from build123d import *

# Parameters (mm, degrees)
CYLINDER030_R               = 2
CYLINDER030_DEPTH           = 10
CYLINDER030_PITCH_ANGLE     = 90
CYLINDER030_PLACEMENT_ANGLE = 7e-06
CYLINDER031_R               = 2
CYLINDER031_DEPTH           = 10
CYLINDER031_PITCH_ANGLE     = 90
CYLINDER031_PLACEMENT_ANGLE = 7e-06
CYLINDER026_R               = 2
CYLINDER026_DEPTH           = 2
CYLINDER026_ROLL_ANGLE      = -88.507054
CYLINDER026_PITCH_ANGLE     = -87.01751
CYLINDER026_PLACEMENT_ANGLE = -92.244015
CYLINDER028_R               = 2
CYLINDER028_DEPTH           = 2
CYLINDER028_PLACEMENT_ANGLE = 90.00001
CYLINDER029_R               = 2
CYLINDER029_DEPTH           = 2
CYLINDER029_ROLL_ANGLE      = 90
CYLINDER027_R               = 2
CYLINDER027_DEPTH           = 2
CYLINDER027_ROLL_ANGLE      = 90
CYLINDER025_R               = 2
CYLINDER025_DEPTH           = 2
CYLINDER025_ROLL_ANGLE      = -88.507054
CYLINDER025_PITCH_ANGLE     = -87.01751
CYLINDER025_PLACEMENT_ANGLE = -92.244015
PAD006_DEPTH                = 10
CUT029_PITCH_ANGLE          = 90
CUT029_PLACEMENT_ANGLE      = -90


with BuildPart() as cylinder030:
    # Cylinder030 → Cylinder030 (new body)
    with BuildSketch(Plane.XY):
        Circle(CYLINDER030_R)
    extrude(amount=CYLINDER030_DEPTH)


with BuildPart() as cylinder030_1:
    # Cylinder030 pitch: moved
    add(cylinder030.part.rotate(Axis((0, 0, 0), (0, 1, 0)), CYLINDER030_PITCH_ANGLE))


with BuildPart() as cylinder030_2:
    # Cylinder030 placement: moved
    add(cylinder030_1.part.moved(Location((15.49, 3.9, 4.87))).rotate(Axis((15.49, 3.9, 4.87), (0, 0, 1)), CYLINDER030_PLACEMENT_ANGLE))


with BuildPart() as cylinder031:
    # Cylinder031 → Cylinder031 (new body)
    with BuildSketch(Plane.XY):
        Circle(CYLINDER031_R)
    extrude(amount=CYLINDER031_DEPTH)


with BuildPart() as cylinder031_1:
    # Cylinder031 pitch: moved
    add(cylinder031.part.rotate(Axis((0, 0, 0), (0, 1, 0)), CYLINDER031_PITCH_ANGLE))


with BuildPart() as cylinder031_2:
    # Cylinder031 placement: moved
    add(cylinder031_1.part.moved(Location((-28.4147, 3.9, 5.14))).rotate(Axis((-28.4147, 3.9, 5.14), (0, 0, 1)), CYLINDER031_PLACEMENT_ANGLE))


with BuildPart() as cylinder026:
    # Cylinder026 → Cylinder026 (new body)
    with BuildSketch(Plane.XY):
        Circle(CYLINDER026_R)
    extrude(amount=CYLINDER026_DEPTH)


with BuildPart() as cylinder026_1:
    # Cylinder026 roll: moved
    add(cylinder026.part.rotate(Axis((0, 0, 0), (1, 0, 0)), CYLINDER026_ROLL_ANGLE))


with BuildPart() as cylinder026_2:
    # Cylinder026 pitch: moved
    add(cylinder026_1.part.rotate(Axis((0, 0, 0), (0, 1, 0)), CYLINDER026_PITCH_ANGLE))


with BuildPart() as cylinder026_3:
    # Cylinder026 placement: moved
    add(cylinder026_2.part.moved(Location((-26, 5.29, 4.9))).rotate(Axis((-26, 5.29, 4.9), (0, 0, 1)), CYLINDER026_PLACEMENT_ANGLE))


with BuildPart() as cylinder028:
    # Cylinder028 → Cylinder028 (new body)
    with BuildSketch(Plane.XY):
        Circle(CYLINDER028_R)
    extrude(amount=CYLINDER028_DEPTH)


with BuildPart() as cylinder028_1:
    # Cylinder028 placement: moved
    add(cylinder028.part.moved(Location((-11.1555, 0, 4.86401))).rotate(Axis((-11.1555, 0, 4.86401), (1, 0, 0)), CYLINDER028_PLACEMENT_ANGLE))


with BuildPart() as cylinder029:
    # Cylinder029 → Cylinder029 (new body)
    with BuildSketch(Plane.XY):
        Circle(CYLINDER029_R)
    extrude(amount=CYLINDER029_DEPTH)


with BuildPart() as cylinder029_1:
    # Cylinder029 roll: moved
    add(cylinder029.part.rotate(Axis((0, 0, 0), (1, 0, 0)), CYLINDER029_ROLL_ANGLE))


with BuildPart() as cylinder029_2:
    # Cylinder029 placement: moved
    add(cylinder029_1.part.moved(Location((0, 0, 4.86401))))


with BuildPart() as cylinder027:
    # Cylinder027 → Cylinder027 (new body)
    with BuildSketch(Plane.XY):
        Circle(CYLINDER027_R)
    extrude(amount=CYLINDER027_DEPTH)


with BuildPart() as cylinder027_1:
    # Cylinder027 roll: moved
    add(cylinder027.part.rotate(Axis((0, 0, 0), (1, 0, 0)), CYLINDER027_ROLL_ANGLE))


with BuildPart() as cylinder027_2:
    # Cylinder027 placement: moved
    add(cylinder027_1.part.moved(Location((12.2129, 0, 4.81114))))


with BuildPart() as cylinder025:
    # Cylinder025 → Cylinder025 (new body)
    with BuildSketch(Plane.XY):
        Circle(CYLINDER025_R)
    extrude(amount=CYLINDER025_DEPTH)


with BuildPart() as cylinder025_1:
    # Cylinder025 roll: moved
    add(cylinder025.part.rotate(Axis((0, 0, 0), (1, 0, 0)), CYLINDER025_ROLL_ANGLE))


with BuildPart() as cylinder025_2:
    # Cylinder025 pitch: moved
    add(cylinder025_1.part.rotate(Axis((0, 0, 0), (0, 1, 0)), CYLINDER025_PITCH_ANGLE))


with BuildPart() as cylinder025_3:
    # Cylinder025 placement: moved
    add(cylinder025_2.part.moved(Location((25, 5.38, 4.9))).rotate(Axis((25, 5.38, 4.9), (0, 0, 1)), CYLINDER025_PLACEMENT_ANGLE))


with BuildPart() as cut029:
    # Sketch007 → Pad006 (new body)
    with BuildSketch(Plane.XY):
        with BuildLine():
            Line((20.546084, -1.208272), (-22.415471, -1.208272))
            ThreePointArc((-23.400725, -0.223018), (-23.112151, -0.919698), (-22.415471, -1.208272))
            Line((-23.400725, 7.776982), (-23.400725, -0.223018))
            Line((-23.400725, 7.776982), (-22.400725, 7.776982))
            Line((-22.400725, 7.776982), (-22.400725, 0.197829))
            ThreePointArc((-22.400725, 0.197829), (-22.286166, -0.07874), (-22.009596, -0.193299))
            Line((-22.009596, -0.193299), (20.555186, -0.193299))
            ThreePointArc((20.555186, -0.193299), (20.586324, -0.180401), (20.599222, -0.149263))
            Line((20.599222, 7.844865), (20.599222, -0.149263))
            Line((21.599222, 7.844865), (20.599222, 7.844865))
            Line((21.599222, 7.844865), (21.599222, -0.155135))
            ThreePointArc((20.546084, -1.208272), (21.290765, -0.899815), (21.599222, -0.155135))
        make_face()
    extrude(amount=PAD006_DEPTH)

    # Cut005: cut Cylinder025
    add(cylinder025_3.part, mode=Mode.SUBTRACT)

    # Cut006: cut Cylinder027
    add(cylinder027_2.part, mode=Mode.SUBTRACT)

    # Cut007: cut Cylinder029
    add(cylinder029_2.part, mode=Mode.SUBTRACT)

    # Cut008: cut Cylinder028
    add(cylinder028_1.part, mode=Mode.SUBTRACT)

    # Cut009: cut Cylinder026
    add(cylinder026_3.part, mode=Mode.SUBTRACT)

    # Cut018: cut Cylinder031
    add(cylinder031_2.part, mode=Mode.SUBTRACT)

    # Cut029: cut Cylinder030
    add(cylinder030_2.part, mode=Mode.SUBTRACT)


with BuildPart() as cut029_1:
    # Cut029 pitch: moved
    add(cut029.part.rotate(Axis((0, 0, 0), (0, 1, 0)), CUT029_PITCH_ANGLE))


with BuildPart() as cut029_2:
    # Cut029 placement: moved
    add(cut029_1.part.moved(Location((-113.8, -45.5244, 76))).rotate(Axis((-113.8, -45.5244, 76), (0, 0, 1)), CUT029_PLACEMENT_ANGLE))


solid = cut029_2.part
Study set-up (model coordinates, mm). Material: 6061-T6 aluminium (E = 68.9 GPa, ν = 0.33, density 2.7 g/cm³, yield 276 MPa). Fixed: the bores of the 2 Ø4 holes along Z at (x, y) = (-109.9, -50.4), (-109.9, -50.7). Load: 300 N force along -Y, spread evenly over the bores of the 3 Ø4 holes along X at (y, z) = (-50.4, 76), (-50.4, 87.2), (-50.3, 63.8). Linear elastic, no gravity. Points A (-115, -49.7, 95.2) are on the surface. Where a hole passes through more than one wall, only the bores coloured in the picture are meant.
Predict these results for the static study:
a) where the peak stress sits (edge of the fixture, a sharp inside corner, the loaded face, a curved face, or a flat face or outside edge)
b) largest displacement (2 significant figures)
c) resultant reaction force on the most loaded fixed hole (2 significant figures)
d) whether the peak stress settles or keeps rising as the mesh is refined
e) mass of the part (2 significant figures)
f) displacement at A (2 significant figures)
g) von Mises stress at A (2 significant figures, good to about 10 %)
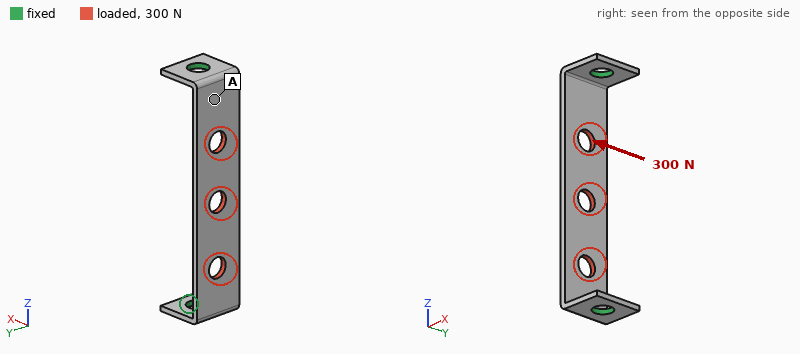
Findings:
a sharp inside corner
80 µm
160 N
keeps rising
1.5 g
21 µm
29 MPa
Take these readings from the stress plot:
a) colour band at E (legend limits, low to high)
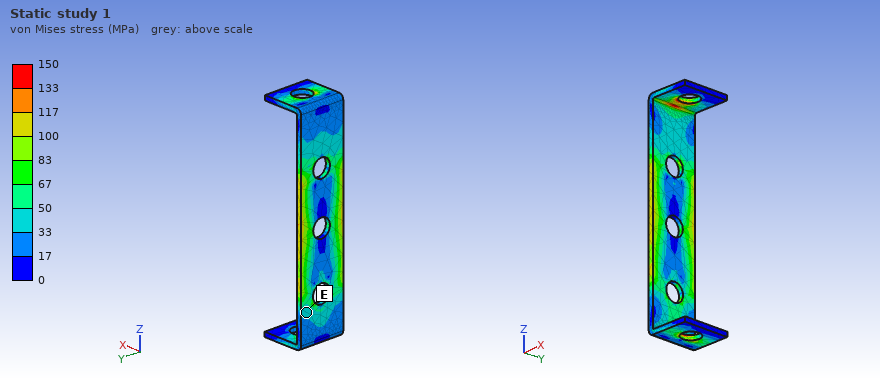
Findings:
33 to 50 MPa
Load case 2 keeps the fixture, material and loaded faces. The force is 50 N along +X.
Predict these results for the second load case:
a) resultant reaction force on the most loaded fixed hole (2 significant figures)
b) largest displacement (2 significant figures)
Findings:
83 N
0.30 mm
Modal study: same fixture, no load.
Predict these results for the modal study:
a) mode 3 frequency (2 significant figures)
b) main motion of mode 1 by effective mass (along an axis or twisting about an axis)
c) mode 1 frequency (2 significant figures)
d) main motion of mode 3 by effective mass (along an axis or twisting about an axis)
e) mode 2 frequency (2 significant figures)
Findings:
7200 Hz
along X
2600 Hz
twisting about Z
6200 Hz
